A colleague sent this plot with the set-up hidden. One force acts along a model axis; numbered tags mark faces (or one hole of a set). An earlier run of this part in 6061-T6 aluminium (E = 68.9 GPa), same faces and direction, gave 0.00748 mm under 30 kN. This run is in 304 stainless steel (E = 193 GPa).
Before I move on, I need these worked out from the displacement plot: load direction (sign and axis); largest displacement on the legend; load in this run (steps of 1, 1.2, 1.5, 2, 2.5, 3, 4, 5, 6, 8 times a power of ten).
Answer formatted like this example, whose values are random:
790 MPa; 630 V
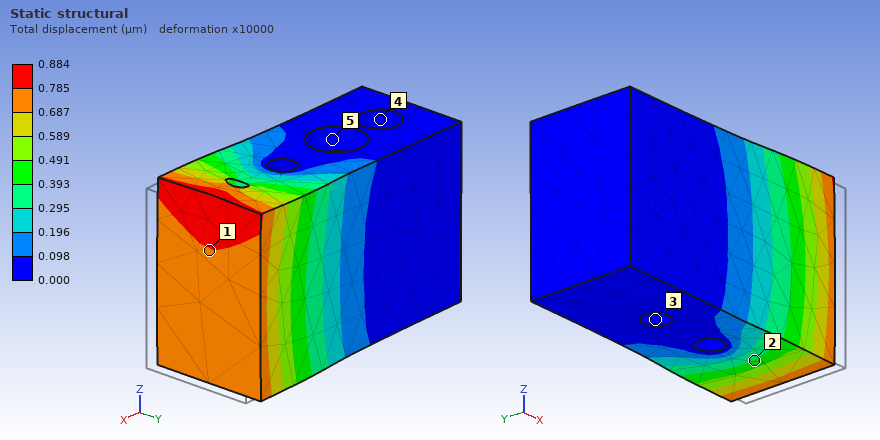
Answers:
-X; 0.884 µm; 10 kN
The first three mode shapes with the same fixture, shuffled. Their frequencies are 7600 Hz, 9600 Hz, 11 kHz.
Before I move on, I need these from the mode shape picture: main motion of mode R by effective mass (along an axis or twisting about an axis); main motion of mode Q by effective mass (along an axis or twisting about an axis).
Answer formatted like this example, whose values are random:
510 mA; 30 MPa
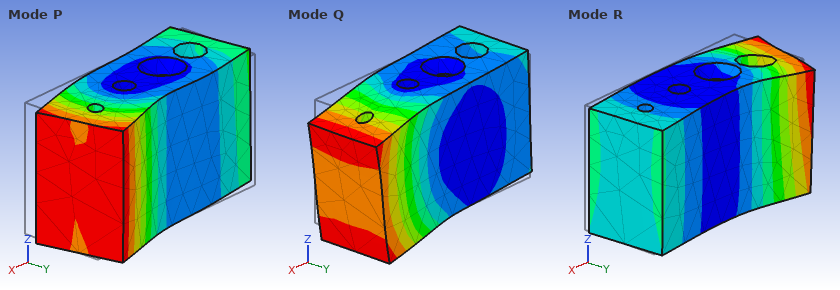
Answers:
along Y; along Z
